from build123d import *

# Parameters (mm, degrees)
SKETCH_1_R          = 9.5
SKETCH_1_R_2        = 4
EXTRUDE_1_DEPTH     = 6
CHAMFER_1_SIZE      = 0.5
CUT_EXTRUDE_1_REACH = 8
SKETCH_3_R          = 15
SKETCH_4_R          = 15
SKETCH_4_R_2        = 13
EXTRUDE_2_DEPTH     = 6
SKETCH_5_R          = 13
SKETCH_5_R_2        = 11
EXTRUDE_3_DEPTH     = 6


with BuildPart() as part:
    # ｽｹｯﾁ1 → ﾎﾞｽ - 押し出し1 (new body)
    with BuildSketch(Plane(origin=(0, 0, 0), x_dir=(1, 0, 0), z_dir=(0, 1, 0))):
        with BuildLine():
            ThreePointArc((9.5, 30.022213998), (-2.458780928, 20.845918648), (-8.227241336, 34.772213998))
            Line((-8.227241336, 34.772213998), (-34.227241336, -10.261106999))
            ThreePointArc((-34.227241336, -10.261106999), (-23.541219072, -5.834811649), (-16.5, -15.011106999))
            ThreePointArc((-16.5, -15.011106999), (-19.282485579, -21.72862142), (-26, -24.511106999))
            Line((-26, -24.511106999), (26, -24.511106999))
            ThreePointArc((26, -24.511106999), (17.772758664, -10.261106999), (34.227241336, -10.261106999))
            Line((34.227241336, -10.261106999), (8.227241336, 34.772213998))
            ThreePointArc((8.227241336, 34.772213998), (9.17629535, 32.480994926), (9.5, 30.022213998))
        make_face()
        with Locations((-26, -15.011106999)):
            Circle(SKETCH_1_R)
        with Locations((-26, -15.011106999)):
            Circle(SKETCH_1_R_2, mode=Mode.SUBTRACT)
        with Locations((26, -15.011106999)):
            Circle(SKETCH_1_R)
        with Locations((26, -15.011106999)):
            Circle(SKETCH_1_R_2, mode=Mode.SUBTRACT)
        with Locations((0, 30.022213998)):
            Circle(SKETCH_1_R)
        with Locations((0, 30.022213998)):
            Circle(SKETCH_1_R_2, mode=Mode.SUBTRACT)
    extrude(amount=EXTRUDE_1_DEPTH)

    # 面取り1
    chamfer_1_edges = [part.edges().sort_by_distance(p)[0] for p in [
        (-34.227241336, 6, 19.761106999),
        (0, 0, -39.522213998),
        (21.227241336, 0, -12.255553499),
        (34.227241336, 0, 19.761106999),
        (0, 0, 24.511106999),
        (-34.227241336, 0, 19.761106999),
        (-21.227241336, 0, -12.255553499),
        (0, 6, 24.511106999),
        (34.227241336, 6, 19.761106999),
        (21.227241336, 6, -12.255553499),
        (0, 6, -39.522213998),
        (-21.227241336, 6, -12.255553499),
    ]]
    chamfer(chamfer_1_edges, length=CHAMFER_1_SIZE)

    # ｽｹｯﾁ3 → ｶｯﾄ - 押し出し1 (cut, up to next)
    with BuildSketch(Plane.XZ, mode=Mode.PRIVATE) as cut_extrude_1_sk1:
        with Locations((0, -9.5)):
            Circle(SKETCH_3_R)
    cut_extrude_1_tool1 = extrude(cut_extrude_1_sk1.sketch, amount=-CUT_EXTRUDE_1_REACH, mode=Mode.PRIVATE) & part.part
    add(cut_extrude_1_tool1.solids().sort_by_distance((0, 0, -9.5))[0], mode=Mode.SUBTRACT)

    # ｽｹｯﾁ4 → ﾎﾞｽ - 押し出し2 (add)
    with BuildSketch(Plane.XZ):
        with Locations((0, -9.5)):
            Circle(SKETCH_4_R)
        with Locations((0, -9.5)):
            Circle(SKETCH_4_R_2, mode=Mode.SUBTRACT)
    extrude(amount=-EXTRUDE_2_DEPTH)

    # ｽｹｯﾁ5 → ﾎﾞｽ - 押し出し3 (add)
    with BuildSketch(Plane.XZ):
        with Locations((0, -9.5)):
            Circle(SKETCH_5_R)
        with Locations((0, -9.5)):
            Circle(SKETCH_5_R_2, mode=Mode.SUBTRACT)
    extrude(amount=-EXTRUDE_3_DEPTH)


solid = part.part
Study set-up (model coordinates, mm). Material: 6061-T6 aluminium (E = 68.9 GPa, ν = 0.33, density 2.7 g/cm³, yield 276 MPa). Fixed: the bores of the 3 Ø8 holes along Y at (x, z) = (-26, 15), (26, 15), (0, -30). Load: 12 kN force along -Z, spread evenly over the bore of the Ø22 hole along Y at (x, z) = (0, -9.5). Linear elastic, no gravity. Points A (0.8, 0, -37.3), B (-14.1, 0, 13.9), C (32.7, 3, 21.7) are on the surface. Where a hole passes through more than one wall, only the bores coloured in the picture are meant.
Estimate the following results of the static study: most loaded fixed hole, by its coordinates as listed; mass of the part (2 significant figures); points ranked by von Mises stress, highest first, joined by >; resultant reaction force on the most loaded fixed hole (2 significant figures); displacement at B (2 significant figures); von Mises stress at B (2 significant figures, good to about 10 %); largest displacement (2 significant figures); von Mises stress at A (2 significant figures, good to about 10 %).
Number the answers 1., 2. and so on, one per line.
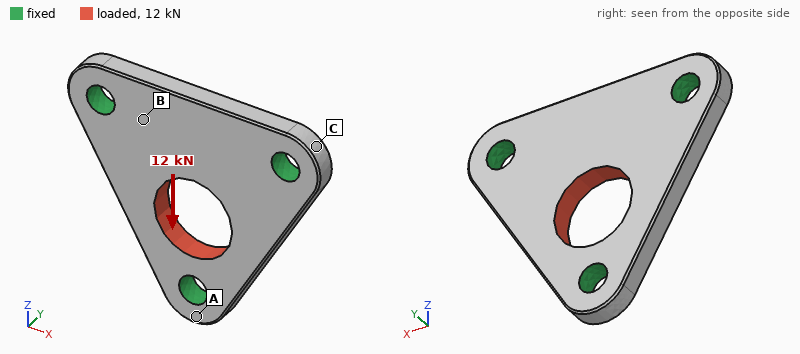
1. (0, -30)
2. 39 g
3. B > A > C
4. 4.8 kN
5. 12 µm
6. 36 MPa
7. 25 µm
8. 20 MPa
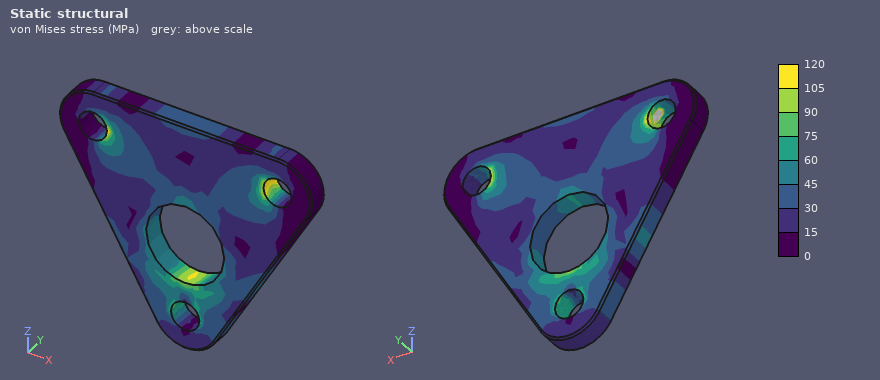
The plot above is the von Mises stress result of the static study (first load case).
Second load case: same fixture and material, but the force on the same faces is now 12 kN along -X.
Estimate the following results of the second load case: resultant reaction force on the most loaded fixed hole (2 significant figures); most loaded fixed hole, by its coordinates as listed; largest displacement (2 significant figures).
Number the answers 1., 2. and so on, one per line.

1. 5.4 kN
2. (0, -30)
3. 26 µm
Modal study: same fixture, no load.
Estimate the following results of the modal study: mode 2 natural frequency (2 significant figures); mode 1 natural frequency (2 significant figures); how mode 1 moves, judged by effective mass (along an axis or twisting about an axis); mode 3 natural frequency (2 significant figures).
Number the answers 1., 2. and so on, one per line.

1. 14 kHz
2. 12 kHz
3. along Y
4. 14 kHz
